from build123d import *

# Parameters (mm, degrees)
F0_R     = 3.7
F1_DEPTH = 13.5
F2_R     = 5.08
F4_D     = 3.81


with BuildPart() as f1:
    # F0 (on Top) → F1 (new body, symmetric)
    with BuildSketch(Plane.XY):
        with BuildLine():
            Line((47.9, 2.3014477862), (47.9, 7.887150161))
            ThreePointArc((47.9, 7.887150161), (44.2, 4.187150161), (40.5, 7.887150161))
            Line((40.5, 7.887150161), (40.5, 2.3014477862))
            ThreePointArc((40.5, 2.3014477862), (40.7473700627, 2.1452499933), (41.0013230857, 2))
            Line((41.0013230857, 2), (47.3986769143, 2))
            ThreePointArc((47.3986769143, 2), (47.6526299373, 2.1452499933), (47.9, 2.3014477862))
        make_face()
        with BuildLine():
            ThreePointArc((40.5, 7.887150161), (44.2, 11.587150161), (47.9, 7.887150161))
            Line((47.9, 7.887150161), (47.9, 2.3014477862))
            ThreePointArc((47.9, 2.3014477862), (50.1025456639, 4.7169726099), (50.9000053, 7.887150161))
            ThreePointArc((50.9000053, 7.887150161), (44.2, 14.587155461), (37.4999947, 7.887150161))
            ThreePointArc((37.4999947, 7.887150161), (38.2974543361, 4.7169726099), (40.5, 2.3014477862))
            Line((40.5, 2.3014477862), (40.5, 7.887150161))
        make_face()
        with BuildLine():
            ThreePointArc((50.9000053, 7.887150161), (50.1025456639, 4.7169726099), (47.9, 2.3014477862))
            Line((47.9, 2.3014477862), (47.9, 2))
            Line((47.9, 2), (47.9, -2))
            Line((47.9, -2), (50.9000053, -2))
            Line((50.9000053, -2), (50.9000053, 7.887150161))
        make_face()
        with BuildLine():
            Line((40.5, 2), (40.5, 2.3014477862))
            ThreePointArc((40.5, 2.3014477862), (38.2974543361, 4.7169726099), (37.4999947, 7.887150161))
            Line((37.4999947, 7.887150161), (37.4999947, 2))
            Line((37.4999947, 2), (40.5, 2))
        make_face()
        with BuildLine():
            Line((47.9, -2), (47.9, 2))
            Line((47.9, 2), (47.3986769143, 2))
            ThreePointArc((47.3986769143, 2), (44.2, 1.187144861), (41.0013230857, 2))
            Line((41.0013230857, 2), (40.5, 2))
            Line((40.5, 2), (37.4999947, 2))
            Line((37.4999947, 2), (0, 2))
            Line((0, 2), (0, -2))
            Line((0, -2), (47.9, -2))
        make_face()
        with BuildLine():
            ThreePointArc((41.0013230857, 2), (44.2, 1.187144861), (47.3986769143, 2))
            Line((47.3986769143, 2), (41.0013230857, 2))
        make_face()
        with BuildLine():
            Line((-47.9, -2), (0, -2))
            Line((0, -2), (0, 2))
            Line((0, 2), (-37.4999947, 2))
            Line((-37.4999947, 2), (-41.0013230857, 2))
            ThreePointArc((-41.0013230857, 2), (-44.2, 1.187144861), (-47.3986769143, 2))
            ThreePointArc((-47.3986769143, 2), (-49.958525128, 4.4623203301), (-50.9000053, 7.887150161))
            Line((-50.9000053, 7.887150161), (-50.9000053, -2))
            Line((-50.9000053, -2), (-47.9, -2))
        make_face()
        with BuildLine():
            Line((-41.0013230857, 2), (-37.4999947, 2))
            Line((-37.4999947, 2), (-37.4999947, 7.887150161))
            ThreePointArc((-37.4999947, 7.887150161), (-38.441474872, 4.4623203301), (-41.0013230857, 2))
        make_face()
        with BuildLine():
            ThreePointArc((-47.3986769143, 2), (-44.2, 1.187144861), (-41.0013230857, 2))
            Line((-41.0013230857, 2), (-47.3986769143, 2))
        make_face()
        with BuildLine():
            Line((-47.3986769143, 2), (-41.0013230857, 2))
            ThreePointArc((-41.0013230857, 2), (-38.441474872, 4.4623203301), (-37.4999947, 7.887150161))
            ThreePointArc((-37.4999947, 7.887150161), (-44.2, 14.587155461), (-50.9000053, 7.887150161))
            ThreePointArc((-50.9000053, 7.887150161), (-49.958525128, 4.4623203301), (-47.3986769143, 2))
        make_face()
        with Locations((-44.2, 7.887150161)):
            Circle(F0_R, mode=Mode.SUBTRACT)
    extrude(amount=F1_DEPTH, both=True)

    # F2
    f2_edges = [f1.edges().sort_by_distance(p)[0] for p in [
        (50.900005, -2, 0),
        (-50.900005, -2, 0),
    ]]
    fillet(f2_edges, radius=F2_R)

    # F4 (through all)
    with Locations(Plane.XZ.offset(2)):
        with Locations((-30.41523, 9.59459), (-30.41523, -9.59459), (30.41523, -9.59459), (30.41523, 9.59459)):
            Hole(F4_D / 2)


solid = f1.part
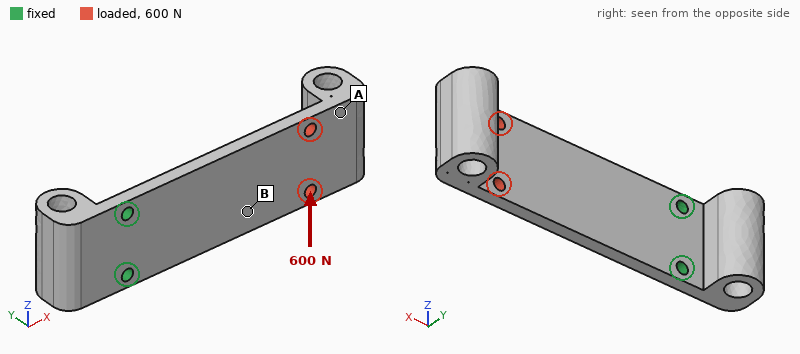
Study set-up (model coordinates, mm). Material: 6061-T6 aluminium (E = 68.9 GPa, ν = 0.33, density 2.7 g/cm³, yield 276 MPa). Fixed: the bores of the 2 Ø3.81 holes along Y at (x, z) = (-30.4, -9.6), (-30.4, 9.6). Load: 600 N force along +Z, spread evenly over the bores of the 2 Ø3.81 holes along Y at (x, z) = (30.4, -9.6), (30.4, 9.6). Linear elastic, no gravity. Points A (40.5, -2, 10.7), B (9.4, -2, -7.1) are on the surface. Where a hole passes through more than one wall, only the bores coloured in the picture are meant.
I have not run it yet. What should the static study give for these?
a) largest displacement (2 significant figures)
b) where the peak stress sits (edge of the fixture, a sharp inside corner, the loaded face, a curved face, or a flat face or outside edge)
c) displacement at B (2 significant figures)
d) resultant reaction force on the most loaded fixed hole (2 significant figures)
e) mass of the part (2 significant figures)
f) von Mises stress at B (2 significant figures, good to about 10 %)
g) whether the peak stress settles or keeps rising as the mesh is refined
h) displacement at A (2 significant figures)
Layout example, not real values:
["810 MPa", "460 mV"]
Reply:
["0.17 mm", "edge of the fixture", "0.060 mm", "1.8 kN", "44 g", "17 MPa", "keeps rising", "0.14 mm"]
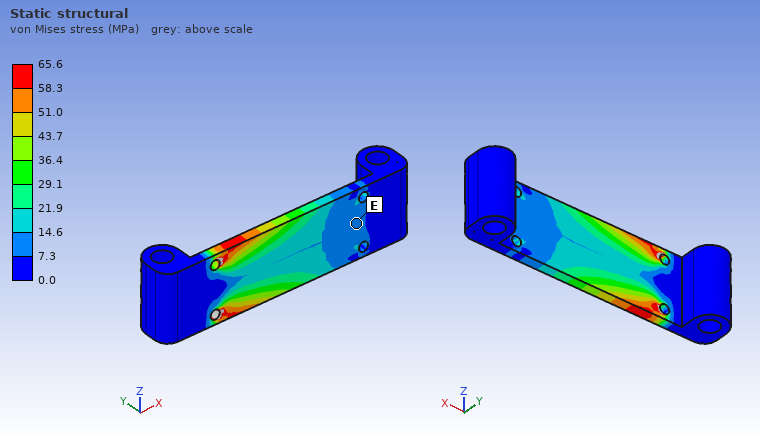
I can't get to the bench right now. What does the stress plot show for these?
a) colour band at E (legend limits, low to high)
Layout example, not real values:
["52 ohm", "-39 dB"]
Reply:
["7.3 to 14.6 MPa"]
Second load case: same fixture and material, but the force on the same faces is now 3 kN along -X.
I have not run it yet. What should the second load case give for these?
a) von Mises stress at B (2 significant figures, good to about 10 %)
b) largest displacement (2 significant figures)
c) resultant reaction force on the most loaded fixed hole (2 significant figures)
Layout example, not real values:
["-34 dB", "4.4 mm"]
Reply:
["28 MPa", "28 µm", "1.5 kN"]
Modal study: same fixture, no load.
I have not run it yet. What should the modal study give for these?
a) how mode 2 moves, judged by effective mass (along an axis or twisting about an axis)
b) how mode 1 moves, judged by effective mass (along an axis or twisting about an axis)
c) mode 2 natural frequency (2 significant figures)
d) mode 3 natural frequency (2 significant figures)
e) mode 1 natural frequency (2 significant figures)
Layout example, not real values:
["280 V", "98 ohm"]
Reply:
["along Z", "along Y", "1700 Hz", "2500 Hz", "350 Hz"]
